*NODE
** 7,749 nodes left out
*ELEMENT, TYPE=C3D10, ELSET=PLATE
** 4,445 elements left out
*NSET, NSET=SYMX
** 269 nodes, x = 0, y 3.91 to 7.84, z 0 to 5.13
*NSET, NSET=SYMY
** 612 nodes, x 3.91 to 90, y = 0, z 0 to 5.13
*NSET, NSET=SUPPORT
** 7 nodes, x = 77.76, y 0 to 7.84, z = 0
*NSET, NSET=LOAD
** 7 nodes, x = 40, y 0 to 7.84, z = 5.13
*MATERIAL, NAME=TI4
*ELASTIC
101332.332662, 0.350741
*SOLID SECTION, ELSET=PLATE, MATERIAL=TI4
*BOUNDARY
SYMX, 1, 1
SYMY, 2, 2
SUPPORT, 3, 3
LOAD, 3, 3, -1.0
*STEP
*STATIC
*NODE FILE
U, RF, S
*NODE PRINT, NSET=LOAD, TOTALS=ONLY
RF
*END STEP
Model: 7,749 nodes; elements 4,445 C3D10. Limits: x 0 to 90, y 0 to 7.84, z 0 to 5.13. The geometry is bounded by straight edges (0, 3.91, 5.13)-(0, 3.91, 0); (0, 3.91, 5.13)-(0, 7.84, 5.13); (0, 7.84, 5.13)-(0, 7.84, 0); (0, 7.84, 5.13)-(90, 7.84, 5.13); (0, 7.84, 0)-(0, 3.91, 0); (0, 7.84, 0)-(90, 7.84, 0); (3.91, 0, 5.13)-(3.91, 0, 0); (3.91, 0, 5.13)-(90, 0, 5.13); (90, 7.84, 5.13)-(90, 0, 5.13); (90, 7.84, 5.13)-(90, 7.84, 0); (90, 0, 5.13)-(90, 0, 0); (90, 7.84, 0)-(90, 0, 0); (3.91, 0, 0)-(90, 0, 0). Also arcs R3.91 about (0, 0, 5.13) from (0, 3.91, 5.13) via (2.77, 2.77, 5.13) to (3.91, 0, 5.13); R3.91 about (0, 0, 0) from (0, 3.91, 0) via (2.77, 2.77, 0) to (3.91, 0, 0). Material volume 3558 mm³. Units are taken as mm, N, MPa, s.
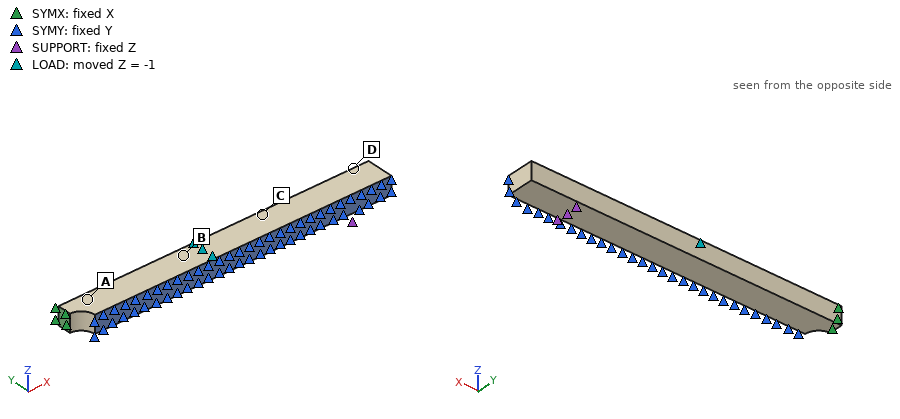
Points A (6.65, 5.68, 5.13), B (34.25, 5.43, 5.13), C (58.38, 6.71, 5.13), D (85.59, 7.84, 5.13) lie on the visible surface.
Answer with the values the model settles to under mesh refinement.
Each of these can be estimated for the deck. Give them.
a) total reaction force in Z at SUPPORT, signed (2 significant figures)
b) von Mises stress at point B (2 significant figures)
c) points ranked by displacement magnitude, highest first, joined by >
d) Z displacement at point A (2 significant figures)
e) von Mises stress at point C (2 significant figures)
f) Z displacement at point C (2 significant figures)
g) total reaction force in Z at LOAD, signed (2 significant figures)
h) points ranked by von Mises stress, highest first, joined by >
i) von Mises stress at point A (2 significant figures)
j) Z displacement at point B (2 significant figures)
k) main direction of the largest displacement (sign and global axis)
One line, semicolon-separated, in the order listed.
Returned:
110 N; 120 MPa; A > B > C > D; -1.4 mm; 62 MPa; -0.56 mm; -110 N; A > B > C > D; 150 MPa; -1.1 mm; -Z
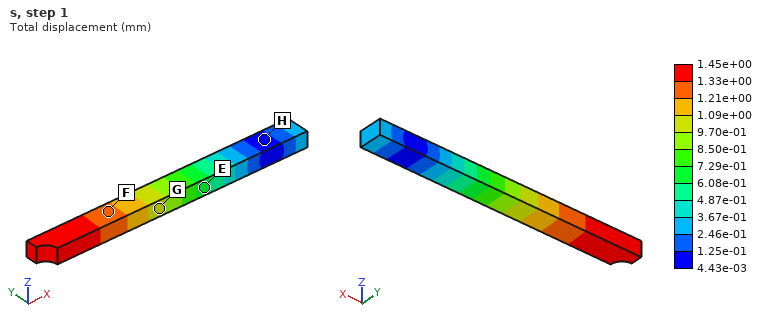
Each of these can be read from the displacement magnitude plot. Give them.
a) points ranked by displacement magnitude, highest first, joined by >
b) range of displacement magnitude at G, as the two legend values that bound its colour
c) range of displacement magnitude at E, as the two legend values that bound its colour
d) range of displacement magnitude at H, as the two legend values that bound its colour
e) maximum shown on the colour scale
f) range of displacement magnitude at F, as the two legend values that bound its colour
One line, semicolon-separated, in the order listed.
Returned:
F > G > E > H; 9.70e-01 to 1.09e+00 mm; 6.08e-01 to 7.29e-01 mm; 4.43e-03 to 1.25e-01 mm; 1.45e+00 mm; 1.21e+00 to 1.33e+00 mm
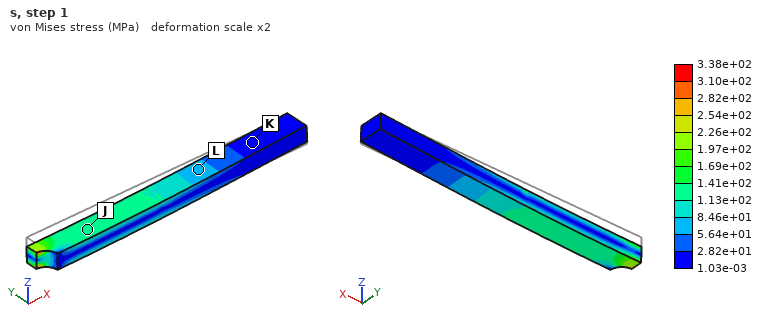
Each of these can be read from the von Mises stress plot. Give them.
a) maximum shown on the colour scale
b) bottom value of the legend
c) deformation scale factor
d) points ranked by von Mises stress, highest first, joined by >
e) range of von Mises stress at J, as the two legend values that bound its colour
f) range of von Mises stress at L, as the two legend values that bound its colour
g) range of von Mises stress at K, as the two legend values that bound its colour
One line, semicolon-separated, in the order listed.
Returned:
3.38e+02 MPa; 1.03e-03 MPa; 2; J > L > K; 1.13e+02 to 1.41e+02 MPa; 5.64e+01 to 8.46e+01 MPa; 1.03e-03 to 2.82e+01 MPa
